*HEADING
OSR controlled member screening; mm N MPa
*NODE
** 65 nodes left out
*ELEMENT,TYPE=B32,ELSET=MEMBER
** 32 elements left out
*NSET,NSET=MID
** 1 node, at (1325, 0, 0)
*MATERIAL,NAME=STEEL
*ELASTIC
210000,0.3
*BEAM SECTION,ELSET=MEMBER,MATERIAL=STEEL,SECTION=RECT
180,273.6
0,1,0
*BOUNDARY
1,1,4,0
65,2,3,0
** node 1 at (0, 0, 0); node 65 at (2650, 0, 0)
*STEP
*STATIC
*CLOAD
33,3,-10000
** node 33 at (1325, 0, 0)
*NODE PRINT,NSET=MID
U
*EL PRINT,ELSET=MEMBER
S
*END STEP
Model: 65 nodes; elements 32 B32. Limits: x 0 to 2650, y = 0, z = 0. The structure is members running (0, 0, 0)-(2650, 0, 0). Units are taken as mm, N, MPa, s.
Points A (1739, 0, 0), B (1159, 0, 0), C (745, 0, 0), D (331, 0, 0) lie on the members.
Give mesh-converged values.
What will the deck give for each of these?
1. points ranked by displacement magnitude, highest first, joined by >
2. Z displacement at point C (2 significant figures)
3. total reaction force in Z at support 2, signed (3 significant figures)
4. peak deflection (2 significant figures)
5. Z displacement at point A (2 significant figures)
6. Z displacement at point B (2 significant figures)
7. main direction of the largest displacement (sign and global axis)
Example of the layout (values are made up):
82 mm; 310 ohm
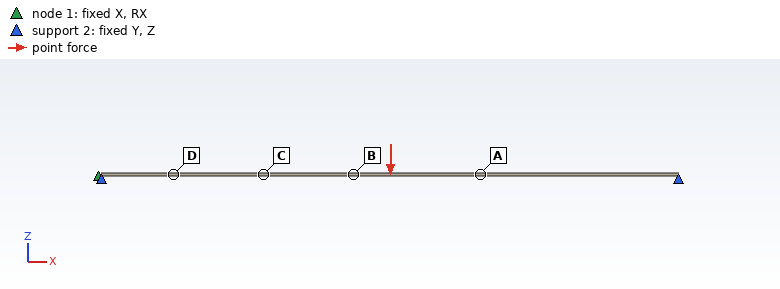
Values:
B > A > C > D; -0.046 mm; 10000 N; 0.062 mm; -0.054 mm; -0.060 mm; -Z
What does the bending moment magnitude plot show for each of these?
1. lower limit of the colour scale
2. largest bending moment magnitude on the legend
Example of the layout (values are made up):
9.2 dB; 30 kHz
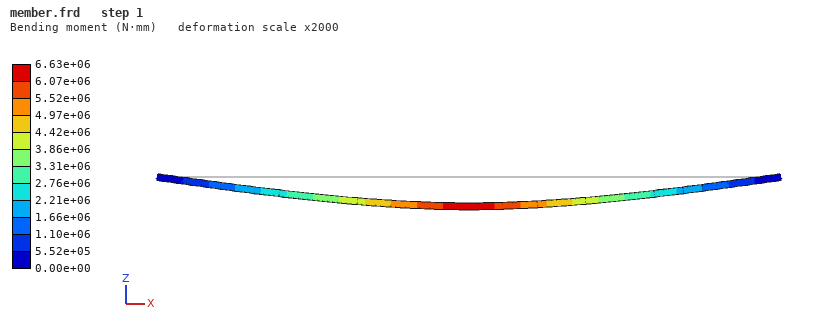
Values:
0.00e+00 N·mm; 6.63e+06 N·mm
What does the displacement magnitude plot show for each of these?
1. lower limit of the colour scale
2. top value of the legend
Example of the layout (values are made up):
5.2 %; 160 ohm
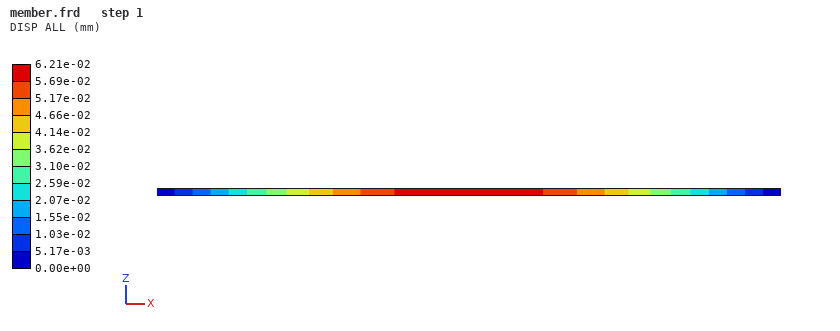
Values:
0.00e+00 mm; 6.21e-02 mm
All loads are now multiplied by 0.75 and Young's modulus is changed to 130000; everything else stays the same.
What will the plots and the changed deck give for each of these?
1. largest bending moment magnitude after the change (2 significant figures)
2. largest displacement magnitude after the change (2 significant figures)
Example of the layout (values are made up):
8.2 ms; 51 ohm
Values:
5.0e+06 N·mm; 0.075 mm
